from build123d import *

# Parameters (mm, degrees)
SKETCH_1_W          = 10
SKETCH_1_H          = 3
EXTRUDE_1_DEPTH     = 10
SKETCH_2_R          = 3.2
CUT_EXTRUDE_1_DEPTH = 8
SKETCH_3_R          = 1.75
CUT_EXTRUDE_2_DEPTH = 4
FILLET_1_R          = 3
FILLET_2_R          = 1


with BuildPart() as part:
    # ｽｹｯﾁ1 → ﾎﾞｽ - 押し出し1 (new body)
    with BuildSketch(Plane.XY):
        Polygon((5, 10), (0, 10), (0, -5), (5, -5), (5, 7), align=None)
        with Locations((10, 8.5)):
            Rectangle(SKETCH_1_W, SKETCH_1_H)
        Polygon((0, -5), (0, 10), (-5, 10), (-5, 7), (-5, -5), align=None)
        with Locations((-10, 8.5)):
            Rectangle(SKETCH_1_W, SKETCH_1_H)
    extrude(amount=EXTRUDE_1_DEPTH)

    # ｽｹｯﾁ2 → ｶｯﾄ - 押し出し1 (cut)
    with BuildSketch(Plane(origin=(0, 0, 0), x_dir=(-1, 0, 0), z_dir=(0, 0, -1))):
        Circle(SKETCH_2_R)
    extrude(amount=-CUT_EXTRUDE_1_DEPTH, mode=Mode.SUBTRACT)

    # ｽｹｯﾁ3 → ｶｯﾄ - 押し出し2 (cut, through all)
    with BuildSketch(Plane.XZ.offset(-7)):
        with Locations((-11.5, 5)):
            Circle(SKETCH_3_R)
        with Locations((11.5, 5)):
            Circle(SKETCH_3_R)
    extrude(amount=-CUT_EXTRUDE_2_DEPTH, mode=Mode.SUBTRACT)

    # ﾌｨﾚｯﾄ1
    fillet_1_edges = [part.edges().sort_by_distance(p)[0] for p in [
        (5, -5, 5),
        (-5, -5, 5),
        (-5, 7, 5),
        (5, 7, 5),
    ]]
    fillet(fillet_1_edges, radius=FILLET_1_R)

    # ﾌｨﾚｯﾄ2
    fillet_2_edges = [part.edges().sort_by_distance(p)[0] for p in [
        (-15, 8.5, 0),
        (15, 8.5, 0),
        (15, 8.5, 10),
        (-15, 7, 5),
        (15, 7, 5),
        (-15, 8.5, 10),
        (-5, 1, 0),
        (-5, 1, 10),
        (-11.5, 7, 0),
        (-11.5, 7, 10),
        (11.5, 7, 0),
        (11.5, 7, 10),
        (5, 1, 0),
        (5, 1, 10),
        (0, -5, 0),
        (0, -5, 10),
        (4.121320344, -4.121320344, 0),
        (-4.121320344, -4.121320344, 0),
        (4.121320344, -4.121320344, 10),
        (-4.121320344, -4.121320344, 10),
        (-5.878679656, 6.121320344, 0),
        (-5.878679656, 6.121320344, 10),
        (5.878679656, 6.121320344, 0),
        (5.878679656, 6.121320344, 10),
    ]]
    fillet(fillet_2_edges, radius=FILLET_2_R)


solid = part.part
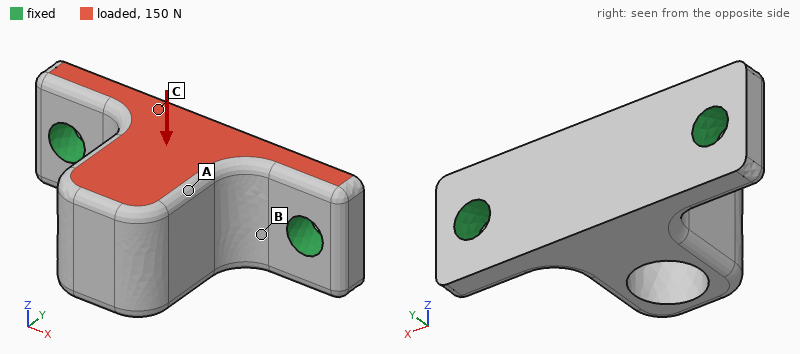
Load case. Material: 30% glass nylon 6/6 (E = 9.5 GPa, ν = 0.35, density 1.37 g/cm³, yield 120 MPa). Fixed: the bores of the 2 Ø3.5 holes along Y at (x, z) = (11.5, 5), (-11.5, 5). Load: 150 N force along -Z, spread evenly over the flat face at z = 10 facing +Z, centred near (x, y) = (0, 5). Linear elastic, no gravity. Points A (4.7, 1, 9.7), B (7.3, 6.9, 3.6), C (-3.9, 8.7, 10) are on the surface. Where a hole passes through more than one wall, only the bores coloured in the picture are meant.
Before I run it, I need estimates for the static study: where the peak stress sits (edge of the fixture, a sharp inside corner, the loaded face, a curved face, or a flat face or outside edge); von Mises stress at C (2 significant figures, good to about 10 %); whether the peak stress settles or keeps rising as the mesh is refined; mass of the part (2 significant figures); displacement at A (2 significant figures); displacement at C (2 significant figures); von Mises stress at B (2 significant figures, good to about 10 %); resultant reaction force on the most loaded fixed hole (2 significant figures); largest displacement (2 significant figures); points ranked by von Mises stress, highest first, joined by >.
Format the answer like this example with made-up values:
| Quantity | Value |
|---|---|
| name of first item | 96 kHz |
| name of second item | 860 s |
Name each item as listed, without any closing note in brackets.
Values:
| Quantity | Value |
|---|---|
| where the peak stress sits | edge of the fixture |
| von Mises stress at C | 5.8 MPa |
| whether the peak stress settles or keeps rising as the mesh is refined | keeps rising |
| mass of the part | 2.4 g |
| displacement at A | 47 µm |
| displacement at C | 22 µm |
| von Mises stress at B | 16 MPa |
| resultant reaction force on the most loaded fixed hole | 75 N |
| largest displacement | 72 µm |
| points ranked by von Mises stress, highest first, joined by > | B > C > A |
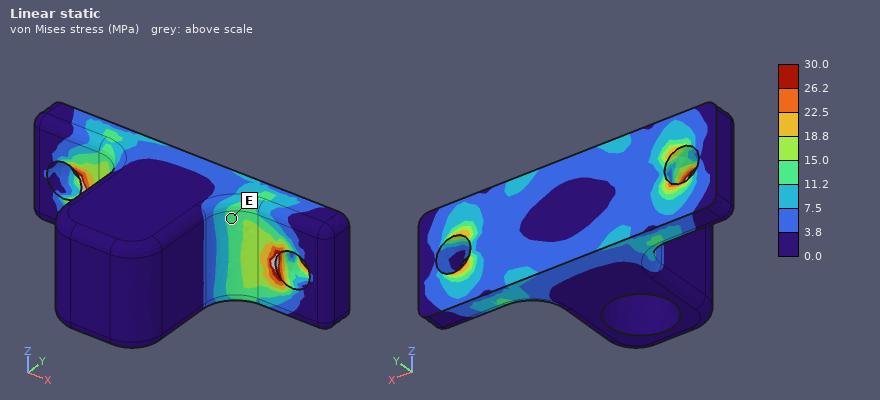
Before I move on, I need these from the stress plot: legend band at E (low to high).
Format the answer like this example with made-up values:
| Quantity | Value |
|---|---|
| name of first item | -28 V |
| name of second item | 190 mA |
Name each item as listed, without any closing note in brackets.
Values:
| Quantity | Value |
|---|---|
| legend band at E | 11.2 to 15.0 MPa |
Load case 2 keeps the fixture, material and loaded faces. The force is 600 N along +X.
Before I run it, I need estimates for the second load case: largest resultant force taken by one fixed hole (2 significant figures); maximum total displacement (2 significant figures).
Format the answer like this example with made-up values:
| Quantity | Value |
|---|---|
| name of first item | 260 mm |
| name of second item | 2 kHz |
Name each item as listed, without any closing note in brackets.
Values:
| Quantity | Value |
|---|---|
| largest resultant force taken by one fixed hole | 350 N |
| maximum total displacement | 59 µm |
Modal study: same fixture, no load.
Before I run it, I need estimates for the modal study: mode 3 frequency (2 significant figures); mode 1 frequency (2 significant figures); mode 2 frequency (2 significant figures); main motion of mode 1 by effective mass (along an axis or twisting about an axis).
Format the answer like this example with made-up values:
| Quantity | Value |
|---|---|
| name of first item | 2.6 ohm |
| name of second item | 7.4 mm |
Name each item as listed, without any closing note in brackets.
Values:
| Quantity | Value |
|---|---|
| mode 3 frequency | 13 kHz |
| mode 1 frequency | 5700 Hz |
| mode 2 frequency | 13 kHz |
| main motion of mode 1 by effective mass | along Z |
